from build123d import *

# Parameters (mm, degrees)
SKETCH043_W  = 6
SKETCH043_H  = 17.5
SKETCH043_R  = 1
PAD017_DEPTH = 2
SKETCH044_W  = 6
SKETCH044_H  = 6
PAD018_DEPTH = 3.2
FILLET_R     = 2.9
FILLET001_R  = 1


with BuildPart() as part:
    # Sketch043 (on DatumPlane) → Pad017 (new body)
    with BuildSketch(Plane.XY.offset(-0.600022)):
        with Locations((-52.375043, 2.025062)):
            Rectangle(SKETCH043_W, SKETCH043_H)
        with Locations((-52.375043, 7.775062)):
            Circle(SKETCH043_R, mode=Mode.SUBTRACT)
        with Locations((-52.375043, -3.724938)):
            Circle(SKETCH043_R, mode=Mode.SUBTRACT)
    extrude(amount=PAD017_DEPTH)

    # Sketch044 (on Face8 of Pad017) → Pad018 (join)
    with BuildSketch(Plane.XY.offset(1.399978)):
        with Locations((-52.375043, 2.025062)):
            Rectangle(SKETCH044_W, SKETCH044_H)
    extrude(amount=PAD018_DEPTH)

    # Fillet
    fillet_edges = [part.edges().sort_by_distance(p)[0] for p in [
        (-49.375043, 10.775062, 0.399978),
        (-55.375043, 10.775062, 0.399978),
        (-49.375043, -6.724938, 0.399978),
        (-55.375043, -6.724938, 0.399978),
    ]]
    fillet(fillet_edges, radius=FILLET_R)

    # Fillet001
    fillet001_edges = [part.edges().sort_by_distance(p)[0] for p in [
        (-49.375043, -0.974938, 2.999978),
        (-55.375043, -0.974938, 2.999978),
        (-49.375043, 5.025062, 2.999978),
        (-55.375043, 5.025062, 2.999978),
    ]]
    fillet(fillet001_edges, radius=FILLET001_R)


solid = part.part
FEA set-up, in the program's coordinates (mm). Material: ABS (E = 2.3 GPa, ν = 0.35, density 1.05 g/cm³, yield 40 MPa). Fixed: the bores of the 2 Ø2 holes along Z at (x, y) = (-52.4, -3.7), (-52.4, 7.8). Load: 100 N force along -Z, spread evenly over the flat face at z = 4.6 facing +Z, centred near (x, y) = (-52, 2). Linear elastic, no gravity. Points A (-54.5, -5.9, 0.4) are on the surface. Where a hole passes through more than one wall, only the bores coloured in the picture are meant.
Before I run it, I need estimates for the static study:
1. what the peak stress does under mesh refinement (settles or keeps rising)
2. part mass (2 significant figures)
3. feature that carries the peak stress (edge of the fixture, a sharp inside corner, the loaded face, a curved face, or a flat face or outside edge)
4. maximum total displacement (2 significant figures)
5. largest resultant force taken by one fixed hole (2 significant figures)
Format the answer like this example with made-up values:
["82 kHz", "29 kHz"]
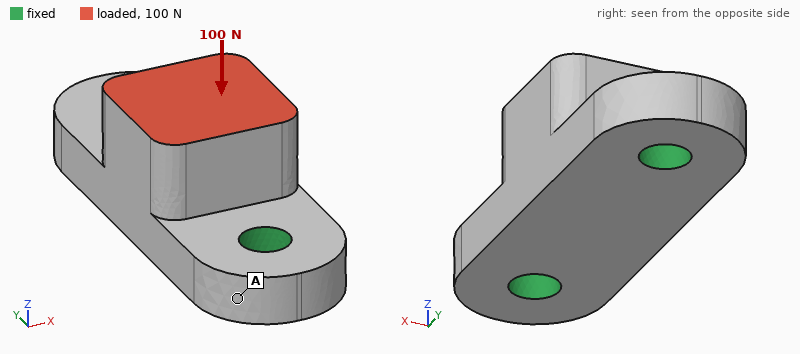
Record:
["keeps rising", "0.31 g", "edge of the fixture", "40 µm", "53 N"]
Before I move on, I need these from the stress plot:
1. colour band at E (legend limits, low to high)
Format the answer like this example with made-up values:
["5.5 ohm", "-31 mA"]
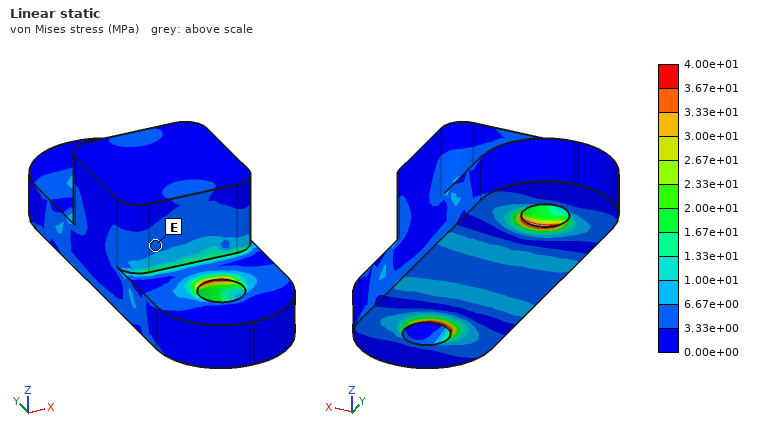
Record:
["3.33e+00 to 6.67e+00 MPa"]
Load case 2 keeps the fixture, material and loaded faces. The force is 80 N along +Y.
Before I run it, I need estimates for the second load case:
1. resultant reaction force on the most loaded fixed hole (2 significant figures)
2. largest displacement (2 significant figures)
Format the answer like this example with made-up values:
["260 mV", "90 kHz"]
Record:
["56 N", "51 µm"]
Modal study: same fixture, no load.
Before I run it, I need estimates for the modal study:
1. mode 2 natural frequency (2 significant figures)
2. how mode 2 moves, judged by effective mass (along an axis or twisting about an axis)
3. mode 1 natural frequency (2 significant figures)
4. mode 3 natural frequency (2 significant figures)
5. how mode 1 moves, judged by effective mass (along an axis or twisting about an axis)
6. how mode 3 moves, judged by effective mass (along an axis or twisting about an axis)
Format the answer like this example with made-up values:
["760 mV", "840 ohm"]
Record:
["18 kHz", "along Z", "12 kHz", "26 kHz", "along X", "along Y"]
